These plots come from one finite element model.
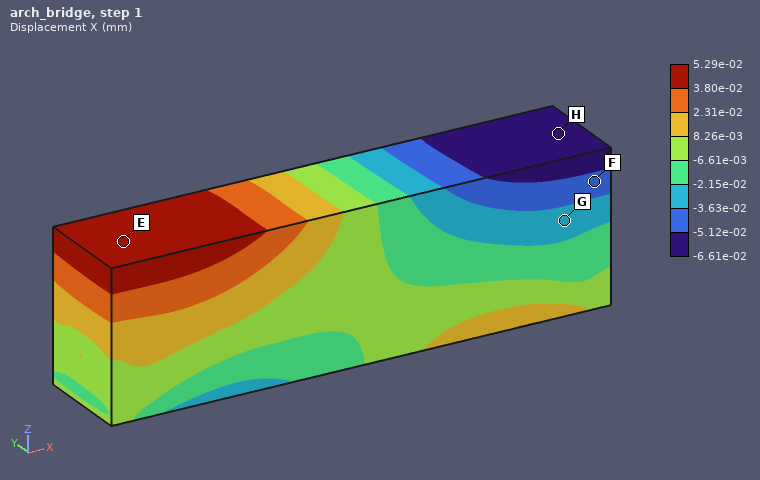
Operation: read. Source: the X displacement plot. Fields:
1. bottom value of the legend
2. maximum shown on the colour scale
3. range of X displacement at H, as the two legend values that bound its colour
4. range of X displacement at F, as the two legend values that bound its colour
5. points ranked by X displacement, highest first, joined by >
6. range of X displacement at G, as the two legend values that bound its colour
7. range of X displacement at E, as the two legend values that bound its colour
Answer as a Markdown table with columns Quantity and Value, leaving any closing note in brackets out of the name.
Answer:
| Quantity | Value |
|---|---|
| bottom value of the legend | -6.61e-02 mm |
| maximum shown on the colour scale | 5.29e-02 mm |
| range of X displacement at H, as the two legend values that bound its colour | -6.61e-02 to -5.12e-02 mm |
| range of X displacement at F, as the two legend values that bound its colour | -5.12e-02 to -3.63e-02 mm |
| points ranked by X displacement, highest first, joined by > | E > G > F > H |
| range of X displacement at G, as the two legend values that bound its colour | -3.63e-02 to -2.15e-02 mm |
| range of X displacement at E, as the two legend values that bound its colour | 3.80e-02 to 5.29e-02 mm |
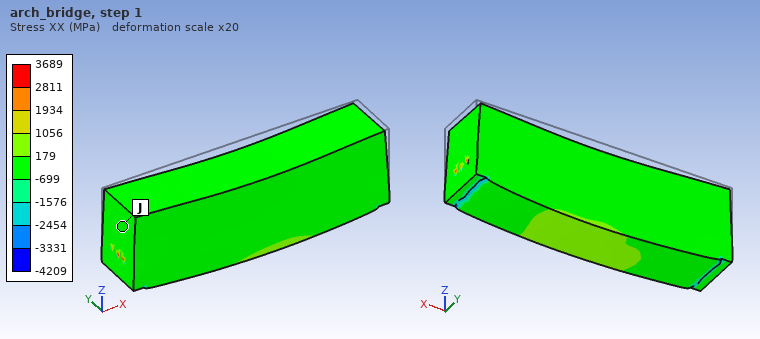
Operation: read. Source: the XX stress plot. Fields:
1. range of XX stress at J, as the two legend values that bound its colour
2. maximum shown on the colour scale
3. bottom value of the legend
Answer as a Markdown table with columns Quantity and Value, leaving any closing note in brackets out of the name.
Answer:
| Quantity | Value |
|---|---|
| range of XX stress at J, as the two legend values that bound its colour | -699 to 179 MPa |
| maximum shown on the colour scale | 3689 MPa |
| bottom value of the legend | -4209 MPa |
